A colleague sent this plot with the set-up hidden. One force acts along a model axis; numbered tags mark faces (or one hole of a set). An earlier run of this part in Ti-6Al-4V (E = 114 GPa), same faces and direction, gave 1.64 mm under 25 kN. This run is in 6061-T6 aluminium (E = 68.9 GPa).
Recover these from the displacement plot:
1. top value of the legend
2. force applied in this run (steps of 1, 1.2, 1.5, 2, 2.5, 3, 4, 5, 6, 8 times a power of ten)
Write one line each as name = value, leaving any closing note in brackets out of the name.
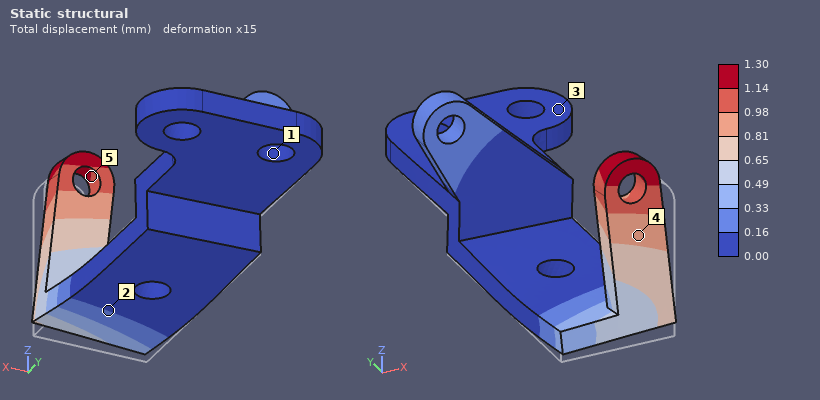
top value of the legend = 1.30 mm
force applied in this run = 12 kN
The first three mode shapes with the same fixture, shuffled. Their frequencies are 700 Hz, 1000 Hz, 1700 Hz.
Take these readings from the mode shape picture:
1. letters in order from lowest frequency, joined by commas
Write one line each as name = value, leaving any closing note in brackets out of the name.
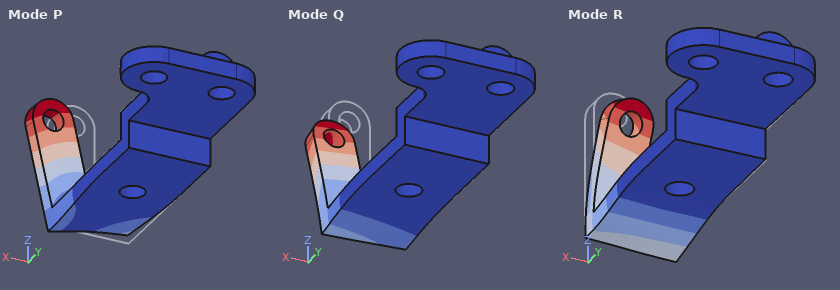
letters in order from lowest frequency, joined by commas = Q, P, R
